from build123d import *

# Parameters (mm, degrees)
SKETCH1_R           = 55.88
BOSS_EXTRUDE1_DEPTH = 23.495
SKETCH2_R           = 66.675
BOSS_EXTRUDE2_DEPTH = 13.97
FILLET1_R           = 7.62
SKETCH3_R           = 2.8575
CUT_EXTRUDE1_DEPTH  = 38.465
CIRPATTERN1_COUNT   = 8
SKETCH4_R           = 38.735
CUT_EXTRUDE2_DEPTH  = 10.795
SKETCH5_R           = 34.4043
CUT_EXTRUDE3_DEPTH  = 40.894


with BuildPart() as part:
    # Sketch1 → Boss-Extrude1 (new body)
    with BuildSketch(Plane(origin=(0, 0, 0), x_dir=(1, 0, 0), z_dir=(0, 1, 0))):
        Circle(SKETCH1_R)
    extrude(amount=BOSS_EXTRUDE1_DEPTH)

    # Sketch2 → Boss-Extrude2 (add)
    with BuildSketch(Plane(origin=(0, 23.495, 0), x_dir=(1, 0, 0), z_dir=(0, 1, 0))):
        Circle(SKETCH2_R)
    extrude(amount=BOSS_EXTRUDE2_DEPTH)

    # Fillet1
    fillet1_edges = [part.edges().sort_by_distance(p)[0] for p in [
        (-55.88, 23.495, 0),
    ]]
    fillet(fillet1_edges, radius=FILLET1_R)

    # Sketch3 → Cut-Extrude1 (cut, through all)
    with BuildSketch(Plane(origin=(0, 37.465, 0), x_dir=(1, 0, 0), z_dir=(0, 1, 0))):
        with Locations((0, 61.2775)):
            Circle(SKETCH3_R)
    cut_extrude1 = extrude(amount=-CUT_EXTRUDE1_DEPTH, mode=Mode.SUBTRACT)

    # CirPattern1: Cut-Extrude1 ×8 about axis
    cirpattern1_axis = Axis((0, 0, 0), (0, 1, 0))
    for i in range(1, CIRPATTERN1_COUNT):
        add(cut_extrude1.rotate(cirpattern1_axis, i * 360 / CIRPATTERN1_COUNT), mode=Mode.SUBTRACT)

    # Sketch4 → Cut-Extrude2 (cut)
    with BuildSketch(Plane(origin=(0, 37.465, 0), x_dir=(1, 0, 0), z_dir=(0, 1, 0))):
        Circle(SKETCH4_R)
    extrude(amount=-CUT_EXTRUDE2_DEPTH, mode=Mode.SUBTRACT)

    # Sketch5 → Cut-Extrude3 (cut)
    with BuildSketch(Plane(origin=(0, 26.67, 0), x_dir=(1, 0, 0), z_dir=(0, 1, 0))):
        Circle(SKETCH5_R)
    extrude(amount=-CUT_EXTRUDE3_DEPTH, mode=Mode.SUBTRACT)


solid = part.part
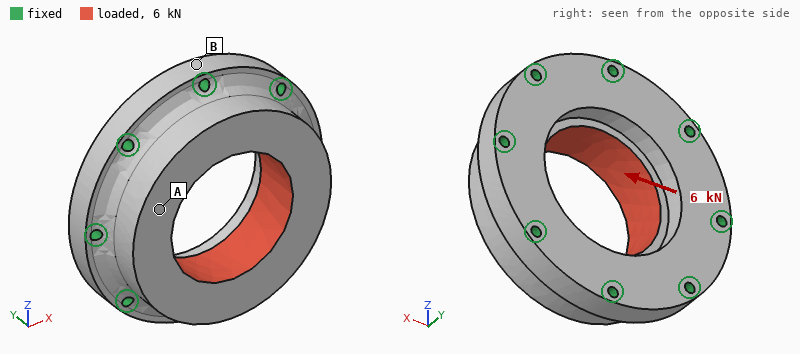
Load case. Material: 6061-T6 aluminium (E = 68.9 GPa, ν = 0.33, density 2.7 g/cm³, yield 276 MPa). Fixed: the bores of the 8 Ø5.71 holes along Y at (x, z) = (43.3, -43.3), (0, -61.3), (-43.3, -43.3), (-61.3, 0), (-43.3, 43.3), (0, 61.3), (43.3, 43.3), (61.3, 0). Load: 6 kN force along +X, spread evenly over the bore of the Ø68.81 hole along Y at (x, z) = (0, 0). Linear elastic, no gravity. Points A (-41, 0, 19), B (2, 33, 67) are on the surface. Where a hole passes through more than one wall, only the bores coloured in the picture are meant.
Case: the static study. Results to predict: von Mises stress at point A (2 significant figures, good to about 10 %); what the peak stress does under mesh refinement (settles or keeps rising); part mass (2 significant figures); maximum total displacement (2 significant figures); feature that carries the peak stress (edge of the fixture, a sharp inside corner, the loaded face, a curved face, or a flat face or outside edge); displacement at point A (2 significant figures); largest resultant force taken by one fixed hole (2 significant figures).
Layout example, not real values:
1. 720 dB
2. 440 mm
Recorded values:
1. 1.9 MPa
2. keeps rising
3. 750 g
4. 2.8 µm
5. edge of the fixture
6. 2.3 µm
7. 960 N
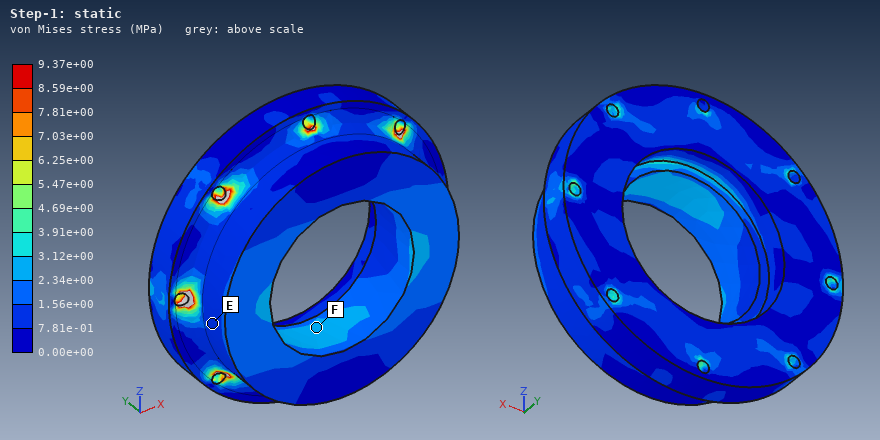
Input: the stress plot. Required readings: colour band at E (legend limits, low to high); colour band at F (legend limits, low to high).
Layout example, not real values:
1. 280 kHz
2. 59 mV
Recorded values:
1. 7.81e-01 to 1.56e+00 MPa
2. 2.34e+00 to 3.12e+00 MPa
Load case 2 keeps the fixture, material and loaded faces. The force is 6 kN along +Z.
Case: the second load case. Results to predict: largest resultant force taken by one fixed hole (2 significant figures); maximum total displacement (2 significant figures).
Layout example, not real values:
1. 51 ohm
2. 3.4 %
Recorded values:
1. 960 N
2. 2.8 µm
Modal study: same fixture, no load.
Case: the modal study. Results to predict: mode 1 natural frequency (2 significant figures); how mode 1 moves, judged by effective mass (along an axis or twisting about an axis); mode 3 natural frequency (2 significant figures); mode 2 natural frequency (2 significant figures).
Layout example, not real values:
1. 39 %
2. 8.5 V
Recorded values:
1. 12 kHz
2. along Y
3. 14 kHz
4. 14 kHz
